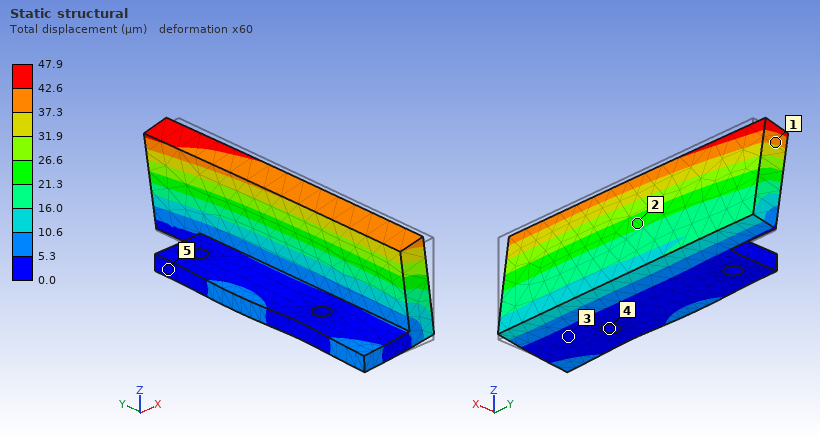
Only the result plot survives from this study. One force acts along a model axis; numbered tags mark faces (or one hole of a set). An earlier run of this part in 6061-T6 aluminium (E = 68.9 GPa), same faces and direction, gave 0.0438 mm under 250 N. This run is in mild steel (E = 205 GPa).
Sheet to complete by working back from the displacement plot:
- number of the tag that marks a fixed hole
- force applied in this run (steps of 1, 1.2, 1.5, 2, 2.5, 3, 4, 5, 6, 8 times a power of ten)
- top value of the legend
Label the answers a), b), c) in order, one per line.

a) 4
b) 800 N
c) 47.9 µm
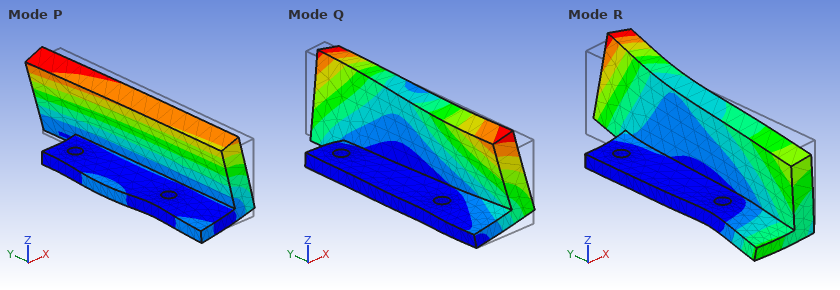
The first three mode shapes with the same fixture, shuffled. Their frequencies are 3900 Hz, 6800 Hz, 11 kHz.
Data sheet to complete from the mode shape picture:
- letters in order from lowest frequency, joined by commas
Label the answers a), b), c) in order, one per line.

a) P, Q, R
